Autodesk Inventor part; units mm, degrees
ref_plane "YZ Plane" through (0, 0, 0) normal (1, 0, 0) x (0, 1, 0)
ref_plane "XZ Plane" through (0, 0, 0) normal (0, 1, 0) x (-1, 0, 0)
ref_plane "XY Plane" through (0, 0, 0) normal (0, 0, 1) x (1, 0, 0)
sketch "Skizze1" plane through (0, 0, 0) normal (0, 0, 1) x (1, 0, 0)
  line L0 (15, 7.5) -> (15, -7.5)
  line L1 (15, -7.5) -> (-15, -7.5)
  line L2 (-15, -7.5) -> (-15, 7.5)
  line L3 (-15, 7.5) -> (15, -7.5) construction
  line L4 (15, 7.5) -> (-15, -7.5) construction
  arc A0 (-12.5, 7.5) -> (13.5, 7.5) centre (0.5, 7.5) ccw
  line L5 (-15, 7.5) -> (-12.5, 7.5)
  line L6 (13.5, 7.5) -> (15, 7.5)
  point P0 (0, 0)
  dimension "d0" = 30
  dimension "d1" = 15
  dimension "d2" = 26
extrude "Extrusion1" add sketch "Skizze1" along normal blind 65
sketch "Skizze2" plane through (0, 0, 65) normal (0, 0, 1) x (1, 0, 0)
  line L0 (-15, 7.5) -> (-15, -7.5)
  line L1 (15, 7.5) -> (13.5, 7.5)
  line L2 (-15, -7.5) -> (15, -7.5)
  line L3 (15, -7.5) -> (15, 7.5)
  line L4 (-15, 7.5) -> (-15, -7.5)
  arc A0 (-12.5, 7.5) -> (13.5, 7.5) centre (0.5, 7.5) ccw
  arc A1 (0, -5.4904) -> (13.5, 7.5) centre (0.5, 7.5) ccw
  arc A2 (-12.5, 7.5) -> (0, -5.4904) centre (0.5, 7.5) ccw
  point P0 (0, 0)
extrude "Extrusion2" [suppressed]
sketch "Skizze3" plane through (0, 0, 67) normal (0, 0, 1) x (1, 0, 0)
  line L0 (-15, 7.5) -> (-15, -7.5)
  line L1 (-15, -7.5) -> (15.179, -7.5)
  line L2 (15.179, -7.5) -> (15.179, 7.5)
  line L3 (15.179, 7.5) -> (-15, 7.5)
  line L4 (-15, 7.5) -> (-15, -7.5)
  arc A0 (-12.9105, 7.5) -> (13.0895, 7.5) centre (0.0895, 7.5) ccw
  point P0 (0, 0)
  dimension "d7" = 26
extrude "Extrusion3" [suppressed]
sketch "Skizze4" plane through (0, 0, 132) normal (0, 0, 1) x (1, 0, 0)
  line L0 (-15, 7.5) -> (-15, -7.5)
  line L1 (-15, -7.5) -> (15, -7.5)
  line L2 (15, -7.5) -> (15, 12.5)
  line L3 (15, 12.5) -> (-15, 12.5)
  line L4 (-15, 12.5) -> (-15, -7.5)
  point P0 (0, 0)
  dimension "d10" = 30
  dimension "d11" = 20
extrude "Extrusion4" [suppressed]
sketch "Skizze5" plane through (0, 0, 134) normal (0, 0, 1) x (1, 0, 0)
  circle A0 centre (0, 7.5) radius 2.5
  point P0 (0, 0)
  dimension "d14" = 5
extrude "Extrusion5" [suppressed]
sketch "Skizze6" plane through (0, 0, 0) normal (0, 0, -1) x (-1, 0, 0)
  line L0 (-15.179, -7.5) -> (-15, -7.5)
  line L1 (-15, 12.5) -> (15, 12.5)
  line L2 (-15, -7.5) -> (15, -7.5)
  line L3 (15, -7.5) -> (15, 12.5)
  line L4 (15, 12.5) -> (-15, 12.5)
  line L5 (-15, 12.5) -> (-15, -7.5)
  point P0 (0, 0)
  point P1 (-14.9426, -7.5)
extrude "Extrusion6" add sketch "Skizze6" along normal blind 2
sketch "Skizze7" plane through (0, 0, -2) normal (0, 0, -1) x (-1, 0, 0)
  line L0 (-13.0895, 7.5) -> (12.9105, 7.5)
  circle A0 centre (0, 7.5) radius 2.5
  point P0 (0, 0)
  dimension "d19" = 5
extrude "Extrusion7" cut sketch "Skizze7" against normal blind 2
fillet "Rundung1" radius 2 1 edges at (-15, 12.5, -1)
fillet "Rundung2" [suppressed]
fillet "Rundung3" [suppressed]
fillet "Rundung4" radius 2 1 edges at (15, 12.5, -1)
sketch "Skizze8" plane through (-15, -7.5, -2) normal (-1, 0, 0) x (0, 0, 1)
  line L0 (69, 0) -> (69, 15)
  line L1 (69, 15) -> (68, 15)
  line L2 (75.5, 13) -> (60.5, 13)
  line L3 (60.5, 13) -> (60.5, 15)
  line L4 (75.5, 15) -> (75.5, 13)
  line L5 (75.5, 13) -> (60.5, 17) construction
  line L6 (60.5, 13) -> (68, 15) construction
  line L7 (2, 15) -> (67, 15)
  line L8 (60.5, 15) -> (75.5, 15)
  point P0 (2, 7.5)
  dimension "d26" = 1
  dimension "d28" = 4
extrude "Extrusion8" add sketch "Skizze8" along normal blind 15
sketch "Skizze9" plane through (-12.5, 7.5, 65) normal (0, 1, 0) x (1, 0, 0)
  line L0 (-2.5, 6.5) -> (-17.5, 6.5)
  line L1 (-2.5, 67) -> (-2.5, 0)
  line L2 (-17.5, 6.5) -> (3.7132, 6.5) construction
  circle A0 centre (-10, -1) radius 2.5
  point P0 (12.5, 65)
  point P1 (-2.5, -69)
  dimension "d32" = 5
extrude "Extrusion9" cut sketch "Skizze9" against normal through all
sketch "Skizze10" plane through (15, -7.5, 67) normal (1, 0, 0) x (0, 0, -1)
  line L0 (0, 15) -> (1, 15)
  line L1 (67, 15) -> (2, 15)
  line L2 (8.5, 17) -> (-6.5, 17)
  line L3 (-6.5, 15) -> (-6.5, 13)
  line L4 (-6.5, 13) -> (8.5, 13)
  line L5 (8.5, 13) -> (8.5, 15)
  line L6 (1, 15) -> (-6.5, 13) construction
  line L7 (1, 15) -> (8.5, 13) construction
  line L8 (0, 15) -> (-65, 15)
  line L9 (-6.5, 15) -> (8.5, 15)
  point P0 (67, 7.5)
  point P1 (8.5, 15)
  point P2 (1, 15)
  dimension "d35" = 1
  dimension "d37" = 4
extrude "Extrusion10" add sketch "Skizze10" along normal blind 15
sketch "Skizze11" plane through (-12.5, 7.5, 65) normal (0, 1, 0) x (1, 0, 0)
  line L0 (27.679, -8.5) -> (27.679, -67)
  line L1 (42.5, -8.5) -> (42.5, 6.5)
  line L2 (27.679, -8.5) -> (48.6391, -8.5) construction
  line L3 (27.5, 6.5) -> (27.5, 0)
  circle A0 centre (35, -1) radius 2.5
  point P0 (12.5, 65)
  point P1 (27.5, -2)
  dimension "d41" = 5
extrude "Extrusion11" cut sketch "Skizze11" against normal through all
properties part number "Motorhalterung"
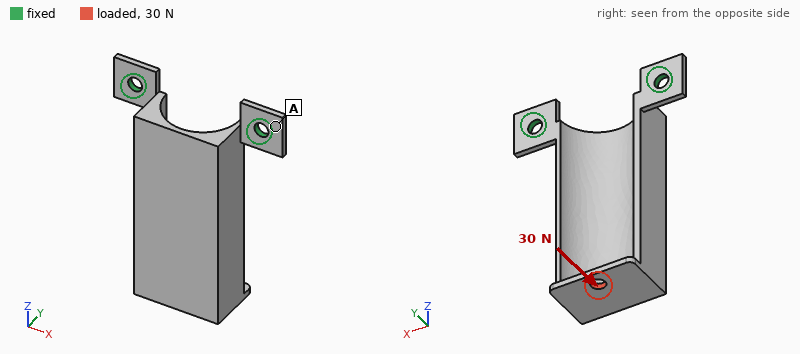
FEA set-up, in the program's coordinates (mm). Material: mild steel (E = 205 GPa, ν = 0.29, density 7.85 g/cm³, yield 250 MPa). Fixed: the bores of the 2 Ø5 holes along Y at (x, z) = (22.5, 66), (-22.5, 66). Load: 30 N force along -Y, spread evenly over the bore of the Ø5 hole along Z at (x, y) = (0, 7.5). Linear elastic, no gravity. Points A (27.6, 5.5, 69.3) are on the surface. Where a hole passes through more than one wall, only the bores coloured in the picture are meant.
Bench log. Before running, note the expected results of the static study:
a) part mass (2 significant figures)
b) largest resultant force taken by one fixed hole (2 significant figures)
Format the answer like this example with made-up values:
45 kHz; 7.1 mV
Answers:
110 g; 24 N
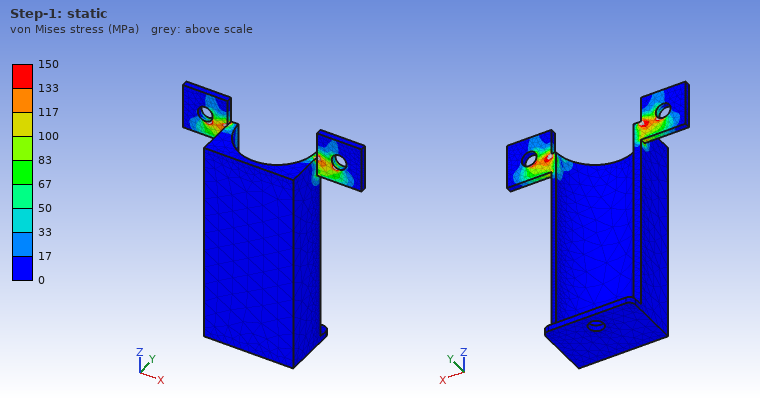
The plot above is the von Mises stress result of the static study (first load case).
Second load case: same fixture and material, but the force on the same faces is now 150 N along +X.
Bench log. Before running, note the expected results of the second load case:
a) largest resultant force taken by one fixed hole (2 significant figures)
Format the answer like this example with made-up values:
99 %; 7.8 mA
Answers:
300 N
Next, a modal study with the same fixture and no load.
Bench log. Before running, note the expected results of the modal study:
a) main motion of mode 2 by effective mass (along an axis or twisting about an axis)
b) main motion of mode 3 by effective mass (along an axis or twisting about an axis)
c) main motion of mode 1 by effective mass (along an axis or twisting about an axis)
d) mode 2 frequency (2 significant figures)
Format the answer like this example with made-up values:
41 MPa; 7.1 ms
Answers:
along X; along X; along Y; 1500 Hz
